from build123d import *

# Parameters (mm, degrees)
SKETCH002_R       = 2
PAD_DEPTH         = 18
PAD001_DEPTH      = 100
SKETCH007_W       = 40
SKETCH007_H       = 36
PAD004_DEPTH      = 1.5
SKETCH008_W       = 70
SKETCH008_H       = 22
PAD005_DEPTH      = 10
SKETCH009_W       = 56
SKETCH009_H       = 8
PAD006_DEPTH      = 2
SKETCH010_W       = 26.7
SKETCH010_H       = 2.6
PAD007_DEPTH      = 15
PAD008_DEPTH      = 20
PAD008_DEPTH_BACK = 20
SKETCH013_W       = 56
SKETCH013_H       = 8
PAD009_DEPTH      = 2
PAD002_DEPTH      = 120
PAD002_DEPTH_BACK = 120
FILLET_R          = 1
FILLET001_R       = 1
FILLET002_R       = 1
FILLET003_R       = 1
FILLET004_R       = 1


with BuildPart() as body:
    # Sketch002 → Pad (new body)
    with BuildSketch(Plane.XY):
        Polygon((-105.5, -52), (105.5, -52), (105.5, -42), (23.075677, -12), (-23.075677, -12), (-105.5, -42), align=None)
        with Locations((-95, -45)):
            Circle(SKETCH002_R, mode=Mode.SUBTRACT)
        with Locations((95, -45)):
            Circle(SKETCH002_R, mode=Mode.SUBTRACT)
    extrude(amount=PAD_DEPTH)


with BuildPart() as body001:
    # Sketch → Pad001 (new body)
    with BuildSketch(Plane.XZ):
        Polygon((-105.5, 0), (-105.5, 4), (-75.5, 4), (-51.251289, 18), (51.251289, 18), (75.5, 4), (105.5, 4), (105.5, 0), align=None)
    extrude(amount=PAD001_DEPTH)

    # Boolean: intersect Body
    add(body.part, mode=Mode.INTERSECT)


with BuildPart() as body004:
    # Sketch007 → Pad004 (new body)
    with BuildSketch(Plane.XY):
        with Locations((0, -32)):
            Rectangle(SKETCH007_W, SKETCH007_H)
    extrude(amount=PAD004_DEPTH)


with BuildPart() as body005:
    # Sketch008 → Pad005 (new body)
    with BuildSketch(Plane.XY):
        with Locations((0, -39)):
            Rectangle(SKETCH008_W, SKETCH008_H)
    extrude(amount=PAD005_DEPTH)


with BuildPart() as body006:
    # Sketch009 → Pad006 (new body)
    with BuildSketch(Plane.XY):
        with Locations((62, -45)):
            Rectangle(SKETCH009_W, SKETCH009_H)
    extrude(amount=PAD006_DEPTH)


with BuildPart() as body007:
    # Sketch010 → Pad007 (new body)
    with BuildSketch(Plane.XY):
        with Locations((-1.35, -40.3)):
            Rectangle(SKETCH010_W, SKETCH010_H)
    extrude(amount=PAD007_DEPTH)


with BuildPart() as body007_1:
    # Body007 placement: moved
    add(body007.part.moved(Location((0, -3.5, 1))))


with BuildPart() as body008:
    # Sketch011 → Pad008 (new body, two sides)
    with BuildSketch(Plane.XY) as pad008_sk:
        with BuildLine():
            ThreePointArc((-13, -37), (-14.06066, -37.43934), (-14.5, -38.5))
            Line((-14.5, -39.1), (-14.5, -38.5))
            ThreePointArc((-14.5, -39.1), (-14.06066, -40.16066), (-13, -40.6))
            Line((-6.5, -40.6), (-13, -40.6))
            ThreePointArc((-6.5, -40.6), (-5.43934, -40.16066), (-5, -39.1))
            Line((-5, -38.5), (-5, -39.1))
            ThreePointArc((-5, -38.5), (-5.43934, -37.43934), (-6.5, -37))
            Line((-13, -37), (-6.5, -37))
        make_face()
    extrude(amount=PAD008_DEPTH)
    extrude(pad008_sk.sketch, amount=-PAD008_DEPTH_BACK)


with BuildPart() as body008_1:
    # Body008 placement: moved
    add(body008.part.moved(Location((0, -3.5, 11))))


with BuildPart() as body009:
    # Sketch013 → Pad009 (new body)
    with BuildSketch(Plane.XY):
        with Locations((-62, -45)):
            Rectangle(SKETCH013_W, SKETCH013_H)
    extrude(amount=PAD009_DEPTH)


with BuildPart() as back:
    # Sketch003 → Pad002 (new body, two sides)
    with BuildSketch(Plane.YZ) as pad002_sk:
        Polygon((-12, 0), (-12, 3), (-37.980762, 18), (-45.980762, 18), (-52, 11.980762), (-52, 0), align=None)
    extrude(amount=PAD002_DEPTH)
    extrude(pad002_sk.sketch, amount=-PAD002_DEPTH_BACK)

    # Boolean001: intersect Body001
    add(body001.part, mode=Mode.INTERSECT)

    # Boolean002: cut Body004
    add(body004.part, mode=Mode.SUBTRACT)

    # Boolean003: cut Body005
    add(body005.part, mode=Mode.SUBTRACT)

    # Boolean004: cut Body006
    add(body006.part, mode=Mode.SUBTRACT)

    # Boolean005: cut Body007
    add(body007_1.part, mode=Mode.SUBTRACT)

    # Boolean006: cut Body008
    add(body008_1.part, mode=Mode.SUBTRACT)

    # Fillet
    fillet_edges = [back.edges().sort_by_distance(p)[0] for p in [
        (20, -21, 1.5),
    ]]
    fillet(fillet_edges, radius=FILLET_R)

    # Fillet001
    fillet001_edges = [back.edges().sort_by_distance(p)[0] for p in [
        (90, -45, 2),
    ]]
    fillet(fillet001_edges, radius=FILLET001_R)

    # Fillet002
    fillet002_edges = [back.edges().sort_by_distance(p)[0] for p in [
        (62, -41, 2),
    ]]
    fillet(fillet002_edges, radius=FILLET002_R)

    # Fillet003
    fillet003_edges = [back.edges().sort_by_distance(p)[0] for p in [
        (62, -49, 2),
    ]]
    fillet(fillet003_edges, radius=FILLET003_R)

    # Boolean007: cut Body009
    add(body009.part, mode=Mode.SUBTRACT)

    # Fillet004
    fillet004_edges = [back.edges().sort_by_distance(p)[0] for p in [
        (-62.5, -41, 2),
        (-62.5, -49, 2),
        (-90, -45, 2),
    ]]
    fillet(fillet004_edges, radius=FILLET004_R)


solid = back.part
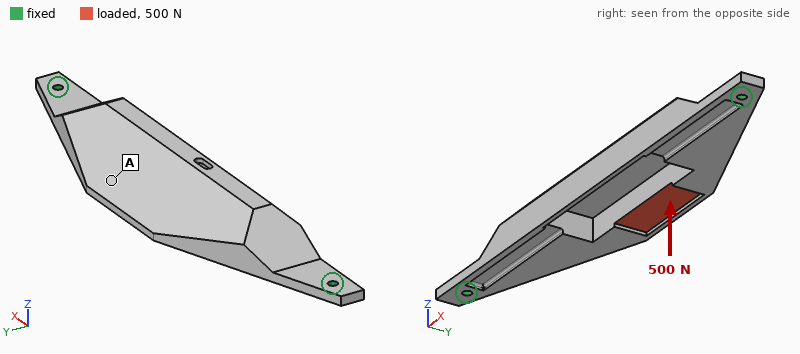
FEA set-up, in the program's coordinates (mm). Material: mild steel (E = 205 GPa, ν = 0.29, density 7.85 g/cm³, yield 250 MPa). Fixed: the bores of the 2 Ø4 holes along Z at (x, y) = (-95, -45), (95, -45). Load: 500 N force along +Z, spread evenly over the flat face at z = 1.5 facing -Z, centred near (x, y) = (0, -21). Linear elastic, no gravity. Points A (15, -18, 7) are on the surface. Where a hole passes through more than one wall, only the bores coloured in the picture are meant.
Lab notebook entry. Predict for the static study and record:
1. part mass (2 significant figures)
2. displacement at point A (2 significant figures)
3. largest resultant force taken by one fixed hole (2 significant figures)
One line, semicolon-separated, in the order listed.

380 g; 0.22 mm; 970 N
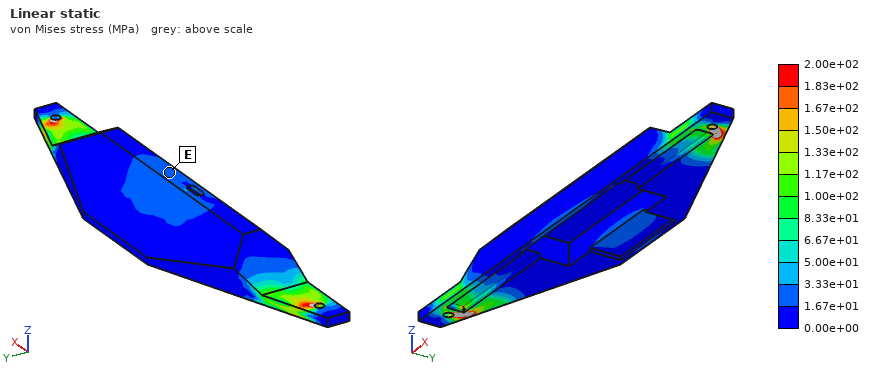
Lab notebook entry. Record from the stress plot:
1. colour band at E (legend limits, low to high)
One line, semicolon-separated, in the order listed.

1.67e+01 to 3.33e+01 MPa
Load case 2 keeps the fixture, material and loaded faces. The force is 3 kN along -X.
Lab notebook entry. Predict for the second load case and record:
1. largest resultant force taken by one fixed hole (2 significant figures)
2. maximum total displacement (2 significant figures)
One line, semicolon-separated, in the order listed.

1.5 kN; 30 µm
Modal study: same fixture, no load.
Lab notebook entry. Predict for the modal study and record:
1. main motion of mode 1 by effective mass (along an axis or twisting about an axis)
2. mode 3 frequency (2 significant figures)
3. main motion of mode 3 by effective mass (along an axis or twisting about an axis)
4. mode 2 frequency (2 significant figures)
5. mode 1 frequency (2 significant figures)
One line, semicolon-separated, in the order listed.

along Z; 2200 Hz; twisting about Y; 1300 Hz; 690 Hz
